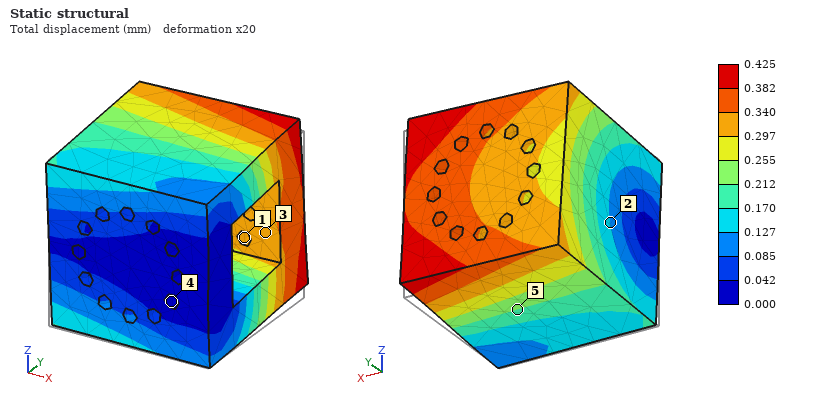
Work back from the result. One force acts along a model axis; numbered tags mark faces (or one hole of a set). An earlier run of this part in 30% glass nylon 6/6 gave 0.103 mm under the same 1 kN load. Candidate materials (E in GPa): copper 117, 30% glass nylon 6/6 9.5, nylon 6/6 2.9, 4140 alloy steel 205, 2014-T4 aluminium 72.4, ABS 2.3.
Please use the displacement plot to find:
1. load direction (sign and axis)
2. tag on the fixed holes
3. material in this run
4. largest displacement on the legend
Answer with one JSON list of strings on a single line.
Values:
["+Z", "4", "ABS", "0.425 mm"]
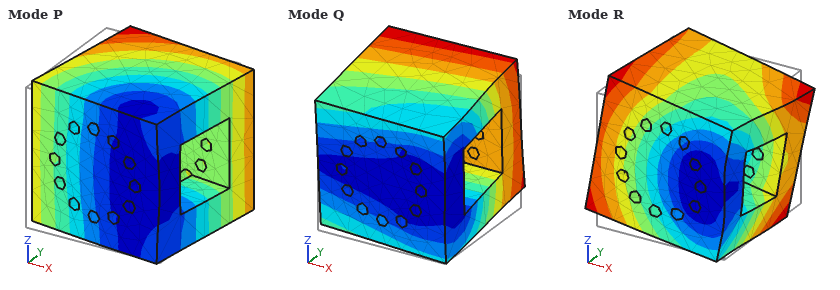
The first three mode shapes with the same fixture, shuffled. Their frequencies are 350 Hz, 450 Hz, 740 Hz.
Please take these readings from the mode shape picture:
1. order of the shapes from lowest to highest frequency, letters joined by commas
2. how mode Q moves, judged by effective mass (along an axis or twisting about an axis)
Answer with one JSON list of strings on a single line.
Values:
["P, Q, R", "along Z"]
